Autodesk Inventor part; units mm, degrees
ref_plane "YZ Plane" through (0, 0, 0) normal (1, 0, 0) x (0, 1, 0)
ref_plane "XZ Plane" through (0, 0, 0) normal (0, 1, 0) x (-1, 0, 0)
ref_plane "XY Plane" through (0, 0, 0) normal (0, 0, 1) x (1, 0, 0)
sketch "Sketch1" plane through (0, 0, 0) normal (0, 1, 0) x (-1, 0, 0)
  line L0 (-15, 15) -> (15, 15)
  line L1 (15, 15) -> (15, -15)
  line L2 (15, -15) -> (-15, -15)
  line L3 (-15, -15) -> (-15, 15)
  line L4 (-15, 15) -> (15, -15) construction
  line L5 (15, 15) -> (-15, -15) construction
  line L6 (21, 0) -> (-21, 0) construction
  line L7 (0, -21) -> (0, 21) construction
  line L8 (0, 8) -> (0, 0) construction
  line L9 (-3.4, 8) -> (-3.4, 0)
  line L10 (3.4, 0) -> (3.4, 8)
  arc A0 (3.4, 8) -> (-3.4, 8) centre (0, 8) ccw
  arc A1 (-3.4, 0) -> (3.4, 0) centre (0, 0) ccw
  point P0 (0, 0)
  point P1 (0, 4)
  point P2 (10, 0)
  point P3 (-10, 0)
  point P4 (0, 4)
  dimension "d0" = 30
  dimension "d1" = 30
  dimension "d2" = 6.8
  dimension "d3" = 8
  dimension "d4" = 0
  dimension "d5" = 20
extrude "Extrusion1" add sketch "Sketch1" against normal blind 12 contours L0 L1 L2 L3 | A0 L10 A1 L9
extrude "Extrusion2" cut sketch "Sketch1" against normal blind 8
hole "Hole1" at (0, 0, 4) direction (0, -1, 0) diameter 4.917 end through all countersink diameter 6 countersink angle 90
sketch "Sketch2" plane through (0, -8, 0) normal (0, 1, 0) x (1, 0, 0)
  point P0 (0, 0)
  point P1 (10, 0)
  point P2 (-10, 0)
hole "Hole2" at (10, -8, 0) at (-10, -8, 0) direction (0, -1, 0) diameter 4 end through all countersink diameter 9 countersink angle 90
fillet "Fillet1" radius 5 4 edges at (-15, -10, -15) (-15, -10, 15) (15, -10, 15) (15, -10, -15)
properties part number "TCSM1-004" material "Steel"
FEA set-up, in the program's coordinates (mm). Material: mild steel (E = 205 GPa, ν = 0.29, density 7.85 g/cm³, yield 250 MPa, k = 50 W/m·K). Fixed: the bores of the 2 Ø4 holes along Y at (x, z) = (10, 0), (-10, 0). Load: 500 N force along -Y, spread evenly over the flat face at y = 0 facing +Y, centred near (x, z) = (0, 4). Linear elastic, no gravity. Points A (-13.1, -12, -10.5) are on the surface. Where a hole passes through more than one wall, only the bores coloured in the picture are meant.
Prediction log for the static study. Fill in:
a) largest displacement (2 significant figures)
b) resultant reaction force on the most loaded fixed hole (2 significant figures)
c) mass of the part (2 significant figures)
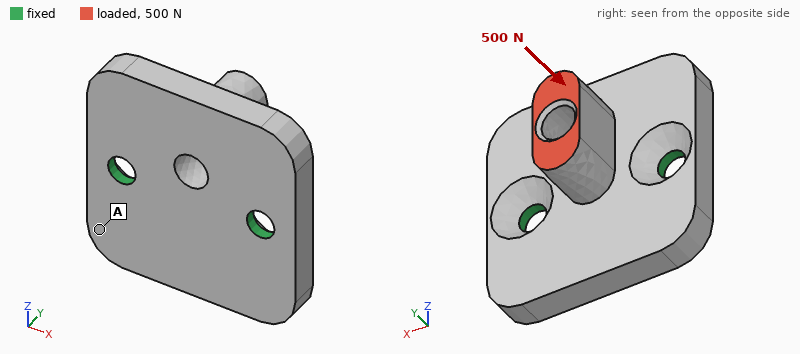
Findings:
9.8 µm
320 N
30 g
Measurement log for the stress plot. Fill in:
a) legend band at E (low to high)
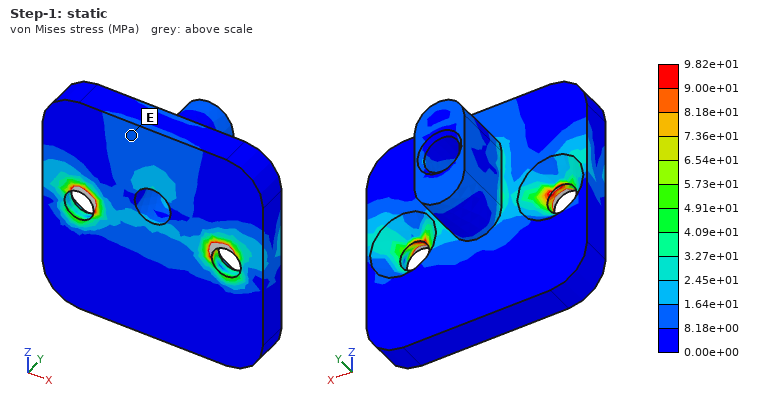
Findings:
8.18e+00 to 1.64e+01 MPa
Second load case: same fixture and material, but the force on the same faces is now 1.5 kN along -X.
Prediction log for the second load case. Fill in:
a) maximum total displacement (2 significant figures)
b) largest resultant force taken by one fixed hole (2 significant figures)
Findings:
21 µm
1.2 kN
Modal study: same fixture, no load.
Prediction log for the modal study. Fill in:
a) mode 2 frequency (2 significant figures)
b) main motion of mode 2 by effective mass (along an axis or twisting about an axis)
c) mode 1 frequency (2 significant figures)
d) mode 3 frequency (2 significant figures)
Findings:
14 kHz
along Y
7000 Hz
18 kHz
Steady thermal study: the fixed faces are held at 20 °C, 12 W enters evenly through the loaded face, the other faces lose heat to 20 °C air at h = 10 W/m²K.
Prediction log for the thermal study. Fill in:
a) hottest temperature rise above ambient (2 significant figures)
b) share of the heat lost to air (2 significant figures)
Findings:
51 K
3.1 %
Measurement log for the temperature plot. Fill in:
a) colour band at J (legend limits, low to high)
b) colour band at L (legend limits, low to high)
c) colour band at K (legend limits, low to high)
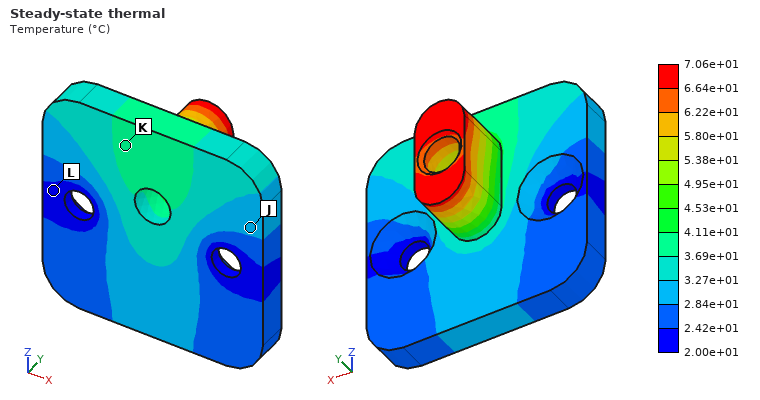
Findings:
2.84e+01 to 3.27e+01 °C
2.00e+01 to 2.42e+01 °C
3.69e+01 to 4.11e+01 °C
